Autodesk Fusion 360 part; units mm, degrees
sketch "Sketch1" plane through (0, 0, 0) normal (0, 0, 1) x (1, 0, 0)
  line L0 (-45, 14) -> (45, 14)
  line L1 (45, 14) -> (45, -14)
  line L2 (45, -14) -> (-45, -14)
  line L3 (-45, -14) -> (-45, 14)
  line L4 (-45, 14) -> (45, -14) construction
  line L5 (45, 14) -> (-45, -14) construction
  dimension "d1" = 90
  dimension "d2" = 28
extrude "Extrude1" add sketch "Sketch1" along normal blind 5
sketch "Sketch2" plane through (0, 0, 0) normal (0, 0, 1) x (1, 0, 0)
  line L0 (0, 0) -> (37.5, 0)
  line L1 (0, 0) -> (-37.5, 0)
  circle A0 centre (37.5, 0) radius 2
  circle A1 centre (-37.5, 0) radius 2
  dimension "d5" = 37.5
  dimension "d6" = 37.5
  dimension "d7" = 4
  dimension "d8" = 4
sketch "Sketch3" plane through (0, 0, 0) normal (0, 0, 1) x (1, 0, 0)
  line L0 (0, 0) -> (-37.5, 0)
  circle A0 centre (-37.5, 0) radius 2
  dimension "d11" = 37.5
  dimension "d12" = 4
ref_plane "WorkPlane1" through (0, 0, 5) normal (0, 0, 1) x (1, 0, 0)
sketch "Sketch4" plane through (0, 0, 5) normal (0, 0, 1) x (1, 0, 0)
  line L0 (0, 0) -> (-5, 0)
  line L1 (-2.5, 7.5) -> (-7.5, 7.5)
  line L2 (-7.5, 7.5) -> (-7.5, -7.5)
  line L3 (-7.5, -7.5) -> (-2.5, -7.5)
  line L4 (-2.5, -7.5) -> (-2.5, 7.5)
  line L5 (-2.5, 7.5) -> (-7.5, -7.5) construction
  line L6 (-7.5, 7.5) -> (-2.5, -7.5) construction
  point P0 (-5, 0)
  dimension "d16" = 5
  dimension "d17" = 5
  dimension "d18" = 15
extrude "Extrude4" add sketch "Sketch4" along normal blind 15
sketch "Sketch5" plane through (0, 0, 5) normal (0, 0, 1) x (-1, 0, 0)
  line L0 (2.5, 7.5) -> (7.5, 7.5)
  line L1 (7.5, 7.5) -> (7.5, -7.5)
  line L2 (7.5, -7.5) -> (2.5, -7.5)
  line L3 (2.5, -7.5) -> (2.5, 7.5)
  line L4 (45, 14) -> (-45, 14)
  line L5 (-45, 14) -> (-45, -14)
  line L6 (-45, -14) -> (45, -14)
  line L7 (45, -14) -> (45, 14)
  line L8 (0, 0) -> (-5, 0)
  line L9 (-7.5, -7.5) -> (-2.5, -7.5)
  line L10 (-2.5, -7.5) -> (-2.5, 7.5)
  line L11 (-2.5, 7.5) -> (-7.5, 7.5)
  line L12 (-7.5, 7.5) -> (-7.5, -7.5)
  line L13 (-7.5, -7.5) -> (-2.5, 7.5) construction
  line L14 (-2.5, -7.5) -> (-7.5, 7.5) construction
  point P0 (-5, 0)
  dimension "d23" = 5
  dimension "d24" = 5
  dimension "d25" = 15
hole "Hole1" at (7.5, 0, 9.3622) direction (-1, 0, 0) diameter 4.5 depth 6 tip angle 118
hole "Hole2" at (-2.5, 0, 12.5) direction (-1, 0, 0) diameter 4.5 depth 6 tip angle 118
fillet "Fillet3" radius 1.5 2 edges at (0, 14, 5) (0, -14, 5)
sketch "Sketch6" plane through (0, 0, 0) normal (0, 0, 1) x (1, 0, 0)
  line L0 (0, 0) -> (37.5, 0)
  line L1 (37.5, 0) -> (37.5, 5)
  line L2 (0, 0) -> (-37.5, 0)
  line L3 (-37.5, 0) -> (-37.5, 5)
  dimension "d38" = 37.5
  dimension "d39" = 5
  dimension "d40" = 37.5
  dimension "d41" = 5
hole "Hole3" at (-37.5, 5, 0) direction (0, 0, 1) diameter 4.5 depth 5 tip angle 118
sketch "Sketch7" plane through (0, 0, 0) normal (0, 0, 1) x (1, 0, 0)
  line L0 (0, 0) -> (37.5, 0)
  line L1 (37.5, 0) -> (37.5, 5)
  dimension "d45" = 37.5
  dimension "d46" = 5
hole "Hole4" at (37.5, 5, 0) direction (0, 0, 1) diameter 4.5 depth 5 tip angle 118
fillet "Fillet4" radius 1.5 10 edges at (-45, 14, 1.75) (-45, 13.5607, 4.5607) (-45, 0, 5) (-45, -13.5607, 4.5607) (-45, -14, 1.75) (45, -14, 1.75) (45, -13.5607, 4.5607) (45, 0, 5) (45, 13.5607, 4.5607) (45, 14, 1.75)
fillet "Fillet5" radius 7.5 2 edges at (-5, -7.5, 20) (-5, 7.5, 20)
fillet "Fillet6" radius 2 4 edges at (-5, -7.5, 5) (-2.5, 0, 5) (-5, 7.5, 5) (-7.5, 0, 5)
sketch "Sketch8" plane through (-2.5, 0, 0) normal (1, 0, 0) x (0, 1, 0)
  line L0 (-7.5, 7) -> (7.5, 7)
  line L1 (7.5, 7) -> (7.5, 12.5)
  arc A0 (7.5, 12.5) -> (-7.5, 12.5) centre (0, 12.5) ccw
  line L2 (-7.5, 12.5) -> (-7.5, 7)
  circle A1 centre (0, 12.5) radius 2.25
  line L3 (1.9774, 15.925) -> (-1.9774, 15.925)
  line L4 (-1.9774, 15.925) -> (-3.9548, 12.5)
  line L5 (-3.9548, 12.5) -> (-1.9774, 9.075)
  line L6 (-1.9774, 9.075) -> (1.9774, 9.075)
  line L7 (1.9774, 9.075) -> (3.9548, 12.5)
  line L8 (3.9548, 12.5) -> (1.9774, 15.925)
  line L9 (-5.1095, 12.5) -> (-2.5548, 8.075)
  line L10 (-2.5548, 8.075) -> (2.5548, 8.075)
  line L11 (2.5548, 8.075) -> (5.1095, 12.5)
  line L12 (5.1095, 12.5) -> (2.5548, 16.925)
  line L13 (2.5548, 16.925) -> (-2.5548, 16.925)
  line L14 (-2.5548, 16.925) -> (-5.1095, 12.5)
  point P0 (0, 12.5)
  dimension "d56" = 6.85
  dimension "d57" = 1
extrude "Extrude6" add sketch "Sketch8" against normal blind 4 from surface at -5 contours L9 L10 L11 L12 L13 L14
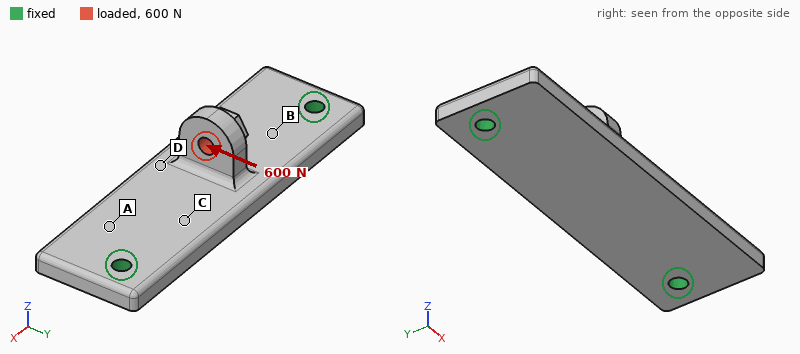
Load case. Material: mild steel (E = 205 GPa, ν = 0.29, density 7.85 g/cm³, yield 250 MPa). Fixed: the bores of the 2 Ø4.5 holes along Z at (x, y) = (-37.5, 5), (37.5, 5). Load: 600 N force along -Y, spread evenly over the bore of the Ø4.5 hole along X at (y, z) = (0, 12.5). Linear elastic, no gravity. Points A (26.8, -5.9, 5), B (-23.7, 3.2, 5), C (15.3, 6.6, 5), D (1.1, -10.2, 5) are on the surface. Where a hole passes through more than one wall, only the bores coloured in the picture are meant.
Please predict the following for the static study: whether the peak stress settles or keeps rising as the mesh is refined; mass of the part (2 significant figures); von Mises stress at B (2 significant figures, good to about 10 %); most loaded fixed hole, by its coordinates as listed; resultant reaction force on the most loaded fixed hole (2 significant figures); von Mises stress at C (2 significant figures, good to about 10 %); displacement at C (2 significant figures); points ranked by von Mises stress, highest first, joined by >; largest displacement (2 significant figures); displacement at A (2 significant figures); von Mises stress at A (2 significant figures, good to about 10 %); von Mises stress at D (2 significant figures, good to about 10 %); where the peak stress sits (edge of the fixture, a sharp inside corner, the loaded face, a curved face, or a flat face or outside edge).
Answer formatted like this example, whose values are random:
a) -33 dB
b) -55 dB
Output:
a) keeps rising
b) 110 g
c) 33 MPa
d) (-37.5, 5)
e) 400 N
f) 25 MPa
g) 4.7 µm
h) B > C > A > D
i) 26 µm
j) 5.1 µm
k) 19 MPa
l) 12 MPa
m) edge of the fixture
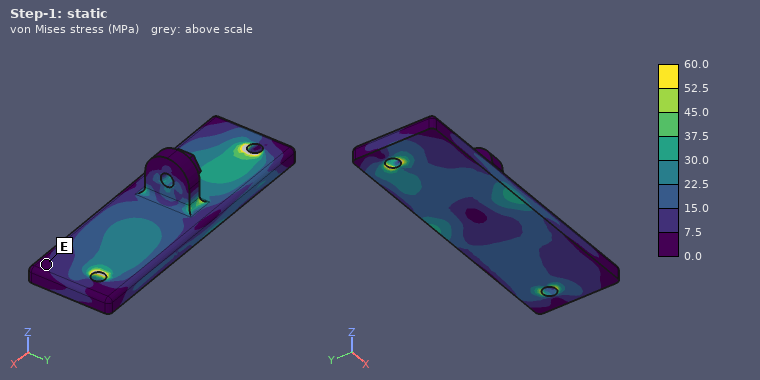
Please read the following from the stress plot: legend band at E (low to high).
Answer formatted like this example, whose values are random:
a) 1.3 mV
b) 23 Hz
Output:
a) 0.0 to 7.5 MPa
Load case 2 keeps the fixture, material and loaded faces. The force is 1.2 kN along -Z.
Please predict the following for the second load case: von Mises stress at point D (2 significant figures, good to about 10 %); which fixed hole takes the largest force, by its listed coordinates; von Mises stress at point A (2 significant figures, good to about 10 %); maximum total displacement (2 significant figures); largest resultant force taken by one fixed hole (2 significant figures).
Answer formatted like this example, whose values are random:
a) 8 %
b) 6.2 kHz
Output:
a) 68 MPa
b) (-37.5, 5)
c) 25 MPa
d) 57 µm
e) 710 N
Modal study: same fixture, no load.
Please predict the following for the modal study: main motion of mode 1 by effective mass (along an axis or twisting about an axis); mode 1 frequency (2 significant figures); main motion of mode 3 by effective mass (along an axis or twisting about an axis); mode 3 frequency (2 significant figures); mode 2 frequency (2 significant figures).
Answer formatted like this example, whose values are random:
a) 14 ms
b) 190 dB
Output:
a) along Z
b) 3700 Hz
c) twisting about Y
d) 9100 Hz
e) 5900 Hz
